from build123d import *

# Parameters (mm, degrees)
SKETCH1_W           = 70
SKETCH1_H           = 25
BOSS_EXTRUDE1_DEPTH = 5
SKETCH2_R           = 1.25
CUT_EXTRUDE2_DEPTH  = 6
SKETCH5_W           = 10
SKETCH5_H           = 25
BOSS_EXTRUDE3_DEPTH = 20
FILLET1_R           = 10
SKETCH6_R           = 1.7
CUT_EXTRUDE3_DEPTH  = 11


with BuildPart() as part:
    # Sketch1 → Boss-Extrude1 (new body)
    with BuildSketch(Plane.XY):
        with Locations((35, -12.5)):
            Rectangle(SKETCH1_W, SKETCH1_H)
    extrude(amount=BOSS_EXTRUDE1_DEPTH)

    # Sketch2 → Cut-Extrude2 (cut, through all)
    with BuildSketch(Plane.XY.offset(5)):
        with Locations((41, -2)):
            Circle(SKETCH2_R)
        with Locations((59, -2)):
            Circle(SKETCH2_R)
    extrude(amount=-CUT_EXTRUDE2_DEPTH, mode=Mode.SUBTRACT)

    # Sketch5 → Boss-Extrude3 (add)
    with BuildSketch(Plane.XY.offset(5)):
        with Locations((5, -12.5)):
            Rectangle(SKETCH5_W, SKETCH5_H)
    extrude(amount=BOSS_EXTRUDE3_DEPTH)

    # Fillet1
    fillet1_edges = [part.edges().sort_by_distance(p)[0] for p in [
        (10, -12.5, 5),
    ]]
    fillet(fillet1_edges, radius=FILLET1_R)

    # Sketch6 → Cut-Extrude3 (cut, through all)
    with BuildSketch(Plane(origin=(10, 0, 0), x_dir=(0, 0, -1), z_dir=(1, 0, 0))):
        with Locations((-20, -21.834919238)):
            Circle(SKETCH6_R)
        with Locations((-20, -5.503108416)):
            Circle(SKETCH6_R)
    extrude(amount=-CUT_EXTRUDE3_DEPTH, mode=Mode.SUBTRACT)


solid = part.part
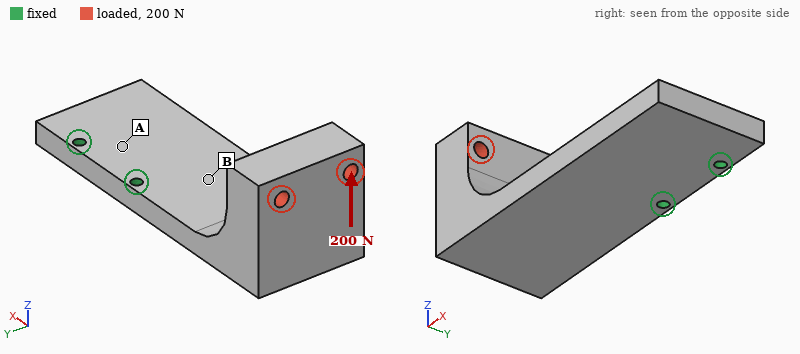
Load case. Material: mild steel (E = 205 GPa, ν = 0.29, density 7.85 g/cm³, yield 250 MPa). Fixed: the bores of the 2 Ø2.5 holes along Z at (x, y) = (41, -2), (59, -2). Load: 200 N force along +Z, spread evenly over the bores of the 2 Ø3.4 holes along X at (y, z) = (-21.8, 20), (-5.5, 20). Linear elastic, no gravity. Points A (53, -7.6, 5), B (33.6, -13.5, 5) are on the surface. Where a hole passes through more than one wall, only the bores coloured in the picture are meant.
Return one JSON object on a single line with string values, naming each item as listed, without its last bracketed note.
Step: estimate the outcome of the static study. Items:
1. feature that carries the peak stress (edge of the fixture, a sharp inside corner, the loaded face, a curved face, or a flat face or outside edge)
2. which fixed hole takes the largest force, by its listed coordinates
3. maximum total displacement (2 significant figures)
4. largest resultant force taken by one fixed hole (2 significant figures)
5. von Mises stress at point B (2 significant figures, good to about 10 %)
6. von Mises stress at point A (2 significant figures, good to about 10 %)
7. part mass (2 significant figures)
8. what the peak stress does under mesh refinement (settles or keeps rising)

{"feature that carries the peak stress": "edge of the fixture", "which fixed hole takes the largest force, by its listed coordinates": "(41, -2)", "maximum total displacement": "0.12 mm", "largest resultant force taken by one fixed hole": "400 N", "von Mises stress at point B": "49 MPa", "von Mises stress at point A": "16 MPa", "part mass": "110 g", "what the peak stress does under mesh refinement": "keeps rising"}
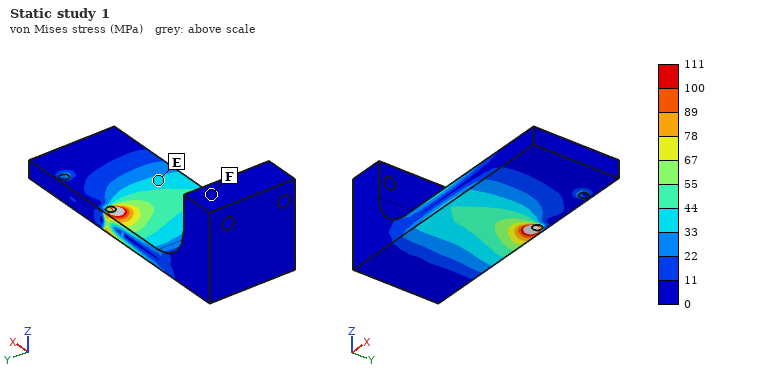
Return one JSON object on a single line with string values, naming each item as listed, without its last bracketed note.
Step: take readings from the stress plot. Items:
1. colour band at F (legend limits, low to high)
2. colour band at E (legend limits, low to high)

{"colour band at F": "0 to 11 MPa", "colour band at E": "33 to 44 MPa"}
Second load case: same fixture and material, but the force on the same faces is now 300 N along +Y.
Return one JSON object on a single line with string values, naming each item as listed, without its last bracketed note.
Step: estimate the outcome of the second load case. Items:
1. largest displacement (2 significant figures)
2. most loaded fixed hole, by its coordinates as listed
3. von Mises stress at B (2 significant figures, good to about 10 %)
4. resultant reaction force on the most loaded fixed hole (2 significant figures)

{"largest displacement": "79 µm", "most loaded fixed hole, by its coordinates as listed": "(41, -2)", "von Mises stress at B": "43 MPa", "resultant reaction force on the most loaded fixed hole": "870 N"}
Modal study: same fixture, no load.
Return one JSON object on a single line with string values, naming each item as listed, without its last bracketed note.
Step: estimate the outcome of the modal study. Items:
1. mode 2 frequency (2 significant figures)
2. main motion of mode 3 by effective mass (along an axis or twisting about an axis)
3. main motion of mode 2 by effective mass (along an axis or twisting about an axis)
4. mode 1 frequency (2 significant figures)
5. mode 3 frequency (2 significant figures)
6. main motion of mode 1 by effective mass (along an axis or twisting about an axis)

{"mode 2 frequency": "2100 Hz", "main motion of mode 3 by effective mass": "along Y", "main motion of mode 2 by effective mass": "along Y", "mode 1 frequency": "970 Hz", "mode 3 frequency": "4500 Hz", "main motion of mode 1 by effective mass": "along Z"}
